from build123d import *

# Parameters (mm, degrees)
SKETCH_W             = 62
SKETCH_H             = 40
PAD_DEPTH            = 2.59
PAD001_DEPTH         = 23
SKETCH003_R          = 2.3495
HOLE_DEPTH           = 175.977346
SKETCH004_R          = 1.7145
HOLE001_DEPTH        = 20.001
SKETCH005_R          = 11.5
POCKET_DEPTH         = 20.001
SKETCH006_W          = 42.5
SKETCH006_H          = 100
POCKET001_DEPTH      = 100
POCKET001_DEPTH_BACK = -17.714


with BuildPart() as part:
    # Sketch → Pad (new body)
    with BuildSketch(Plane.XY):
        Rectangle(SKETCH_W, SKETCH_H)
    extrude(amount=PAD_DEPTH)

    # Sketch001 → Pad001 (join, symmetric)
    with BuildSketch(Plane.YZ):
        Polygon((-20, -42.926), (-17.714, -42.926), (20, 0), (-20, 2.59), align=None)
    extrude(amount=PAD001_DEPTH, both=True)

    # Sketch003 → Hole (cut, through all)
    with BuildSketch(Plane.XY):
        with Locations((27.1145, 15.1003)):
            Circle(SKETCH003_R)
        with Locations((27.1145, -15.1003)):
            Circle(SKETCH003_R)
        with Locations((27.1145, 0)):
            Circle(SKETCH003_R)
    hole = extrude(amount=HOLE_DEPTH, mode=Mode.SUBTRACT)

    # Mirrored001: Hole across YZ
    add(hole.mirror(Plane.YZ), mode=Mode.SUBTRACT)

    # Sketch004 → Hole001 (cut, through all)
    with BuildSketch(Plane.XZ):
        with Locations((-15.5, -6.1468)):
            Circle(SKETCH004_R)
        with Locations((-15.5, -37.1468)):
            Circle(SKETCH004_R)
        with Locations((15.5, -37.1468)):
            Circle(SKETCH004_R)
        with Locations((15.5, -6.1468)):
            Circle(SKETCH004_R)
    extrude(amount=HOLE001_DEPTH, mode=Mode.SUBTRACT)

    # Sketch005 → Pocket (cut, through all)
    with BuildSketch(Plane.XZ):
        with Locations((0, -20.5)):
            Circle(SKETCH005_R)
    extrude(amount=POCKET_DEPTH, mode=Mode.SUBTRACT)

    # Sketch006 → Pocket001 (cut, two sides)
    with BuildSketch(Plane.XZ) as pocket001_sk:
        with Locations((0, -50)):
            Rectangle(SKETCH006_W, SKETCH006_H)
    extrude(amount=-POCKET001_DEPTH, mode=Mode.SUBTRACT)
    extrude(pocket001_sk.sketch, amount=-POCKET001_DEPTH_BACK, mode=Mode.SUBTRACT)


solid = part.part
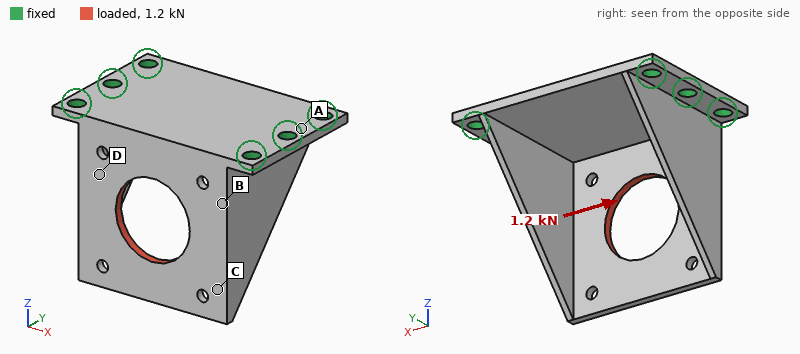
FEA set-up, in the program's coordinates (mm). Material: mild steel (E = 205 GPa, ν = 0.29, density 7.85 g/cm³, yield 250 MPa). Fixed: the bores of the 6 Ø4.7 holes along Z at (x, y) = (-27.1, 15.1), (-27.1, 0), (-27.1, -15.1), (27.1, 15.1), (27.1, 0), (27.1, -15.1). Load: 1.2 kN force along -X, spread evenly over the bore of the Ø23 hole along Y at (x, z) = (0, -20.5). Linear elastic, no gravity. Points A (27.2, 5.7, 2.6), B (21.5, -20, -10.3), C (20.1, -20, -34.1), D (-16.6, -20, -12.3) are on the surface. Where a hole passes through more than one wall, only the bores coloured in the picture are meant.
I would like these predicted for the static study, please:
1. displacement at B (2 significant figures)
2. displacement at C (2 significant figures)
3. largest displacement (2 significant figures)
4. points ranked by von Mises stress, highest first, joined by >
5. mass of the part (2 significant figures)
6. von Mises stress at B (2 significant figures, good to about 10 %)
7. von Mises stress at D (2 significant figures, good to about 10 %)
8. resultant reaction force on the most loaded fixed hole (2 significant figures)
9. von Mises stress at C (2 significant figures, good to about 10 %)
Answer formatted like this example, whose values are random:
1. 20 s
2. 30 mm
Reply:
1. 5.8 µm
2. 16 µm
3. 19 µm
4. D > B > C > A
5. 98 g
6. 21 MPa
7. 25 MPa
8. 710 N
9. 10 MPa
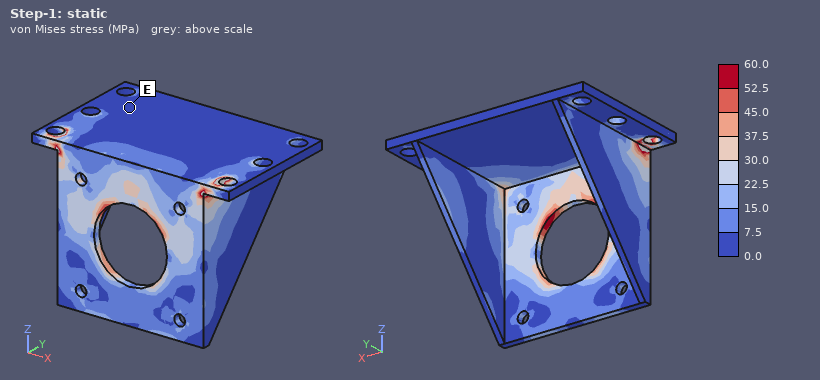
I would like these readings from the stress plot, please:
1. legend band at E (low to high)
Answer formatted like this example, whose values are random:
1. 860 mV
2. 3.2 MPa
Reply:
1. 0.0 to 7.5 MPa
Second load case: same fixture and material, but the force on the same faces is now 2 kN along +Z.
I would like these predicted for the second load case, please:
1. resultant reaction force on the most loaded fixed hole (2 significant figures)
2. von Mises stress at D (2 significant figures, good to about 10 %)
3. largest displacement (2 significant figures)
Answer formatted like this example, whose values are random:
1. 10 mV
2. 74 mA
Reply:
1. 1.1 kN
2. 31 MPa
3. 22 µm
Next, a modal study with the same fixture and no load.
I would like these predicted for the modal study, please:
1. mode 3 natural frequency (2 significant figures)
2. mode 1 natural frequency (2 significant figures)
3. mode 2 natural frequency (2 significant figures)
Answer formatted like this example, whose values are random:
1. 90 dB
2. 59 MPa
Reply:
1. 5600 Hz
2. 3400 Hz
3. 5500 Hz
